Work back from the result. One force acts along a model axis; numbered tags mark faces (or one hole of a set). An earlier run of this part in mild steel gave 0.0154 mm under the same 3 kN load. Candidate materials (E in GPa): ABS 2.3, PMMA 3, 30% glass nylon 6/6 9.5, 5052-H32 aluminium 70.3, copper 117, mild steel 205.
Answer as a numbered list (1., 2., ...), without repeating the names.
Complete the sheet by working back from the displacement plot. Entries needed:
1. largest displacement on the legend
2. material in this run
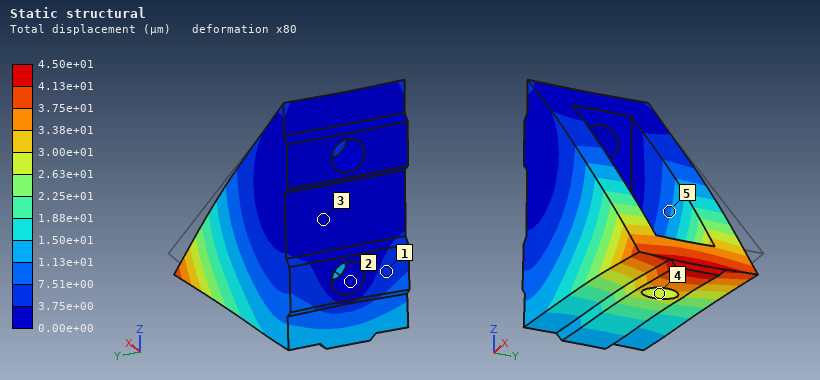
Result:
1. 4.50e+01 µm
2. 5052-H32 aluminium
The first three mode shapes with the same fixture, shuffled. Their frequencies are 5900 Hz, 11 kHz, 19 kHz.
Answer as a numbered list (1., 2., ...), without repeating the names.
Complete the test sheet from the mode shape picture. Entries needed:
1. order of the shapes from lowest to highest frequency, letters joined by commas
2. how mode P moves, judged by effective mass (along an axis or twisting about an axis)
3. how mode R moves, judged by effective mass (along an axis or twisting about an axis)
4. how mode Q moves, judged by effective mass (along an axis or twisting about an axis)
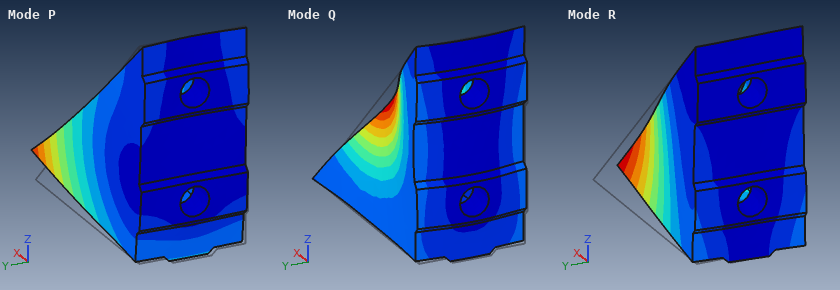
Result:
1. R, P, Q
2. along Z
3. along Y
4. along X
